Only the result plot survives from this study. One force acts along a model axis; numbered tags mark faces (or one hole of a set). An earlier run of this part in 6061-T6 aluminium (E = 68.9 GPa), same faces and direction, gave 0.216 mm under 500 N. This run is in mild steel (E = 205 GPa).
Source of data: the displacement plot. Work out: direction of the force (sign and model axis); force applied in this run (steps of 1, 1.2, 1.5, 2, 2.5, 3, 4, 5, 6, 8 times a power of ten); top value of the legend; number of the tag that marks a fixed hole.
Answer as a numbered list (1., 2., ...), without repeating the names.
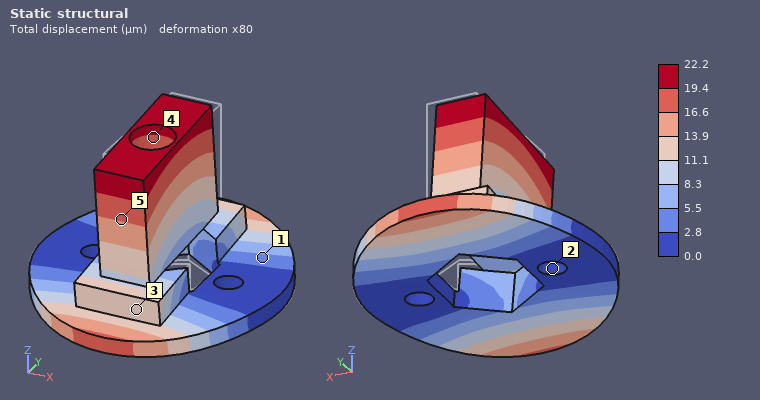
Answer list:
1. -Y
2. 150 N
3. 22.2 µm
4. 2
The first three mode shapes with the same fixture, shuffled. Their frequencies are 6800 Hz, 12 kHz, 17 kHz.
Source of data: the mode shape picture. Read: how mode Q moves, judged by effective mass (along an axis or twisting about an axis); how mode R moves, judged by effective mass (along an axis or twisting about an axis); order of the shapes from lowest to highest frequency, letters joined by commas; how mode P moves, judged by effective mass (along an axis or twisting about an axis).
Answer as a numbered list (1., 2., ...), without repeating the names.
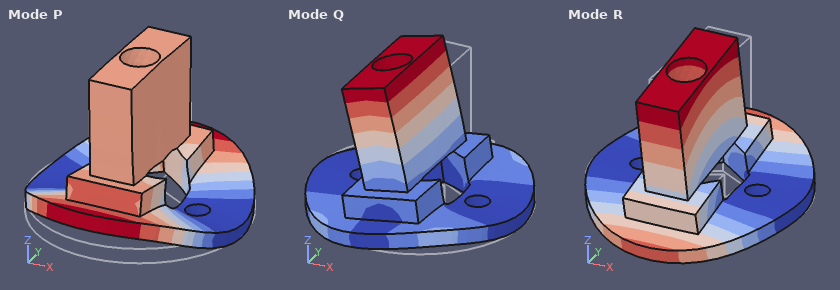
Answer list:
1. along X
2. along Y
3. R, Q, P
4. along Z
